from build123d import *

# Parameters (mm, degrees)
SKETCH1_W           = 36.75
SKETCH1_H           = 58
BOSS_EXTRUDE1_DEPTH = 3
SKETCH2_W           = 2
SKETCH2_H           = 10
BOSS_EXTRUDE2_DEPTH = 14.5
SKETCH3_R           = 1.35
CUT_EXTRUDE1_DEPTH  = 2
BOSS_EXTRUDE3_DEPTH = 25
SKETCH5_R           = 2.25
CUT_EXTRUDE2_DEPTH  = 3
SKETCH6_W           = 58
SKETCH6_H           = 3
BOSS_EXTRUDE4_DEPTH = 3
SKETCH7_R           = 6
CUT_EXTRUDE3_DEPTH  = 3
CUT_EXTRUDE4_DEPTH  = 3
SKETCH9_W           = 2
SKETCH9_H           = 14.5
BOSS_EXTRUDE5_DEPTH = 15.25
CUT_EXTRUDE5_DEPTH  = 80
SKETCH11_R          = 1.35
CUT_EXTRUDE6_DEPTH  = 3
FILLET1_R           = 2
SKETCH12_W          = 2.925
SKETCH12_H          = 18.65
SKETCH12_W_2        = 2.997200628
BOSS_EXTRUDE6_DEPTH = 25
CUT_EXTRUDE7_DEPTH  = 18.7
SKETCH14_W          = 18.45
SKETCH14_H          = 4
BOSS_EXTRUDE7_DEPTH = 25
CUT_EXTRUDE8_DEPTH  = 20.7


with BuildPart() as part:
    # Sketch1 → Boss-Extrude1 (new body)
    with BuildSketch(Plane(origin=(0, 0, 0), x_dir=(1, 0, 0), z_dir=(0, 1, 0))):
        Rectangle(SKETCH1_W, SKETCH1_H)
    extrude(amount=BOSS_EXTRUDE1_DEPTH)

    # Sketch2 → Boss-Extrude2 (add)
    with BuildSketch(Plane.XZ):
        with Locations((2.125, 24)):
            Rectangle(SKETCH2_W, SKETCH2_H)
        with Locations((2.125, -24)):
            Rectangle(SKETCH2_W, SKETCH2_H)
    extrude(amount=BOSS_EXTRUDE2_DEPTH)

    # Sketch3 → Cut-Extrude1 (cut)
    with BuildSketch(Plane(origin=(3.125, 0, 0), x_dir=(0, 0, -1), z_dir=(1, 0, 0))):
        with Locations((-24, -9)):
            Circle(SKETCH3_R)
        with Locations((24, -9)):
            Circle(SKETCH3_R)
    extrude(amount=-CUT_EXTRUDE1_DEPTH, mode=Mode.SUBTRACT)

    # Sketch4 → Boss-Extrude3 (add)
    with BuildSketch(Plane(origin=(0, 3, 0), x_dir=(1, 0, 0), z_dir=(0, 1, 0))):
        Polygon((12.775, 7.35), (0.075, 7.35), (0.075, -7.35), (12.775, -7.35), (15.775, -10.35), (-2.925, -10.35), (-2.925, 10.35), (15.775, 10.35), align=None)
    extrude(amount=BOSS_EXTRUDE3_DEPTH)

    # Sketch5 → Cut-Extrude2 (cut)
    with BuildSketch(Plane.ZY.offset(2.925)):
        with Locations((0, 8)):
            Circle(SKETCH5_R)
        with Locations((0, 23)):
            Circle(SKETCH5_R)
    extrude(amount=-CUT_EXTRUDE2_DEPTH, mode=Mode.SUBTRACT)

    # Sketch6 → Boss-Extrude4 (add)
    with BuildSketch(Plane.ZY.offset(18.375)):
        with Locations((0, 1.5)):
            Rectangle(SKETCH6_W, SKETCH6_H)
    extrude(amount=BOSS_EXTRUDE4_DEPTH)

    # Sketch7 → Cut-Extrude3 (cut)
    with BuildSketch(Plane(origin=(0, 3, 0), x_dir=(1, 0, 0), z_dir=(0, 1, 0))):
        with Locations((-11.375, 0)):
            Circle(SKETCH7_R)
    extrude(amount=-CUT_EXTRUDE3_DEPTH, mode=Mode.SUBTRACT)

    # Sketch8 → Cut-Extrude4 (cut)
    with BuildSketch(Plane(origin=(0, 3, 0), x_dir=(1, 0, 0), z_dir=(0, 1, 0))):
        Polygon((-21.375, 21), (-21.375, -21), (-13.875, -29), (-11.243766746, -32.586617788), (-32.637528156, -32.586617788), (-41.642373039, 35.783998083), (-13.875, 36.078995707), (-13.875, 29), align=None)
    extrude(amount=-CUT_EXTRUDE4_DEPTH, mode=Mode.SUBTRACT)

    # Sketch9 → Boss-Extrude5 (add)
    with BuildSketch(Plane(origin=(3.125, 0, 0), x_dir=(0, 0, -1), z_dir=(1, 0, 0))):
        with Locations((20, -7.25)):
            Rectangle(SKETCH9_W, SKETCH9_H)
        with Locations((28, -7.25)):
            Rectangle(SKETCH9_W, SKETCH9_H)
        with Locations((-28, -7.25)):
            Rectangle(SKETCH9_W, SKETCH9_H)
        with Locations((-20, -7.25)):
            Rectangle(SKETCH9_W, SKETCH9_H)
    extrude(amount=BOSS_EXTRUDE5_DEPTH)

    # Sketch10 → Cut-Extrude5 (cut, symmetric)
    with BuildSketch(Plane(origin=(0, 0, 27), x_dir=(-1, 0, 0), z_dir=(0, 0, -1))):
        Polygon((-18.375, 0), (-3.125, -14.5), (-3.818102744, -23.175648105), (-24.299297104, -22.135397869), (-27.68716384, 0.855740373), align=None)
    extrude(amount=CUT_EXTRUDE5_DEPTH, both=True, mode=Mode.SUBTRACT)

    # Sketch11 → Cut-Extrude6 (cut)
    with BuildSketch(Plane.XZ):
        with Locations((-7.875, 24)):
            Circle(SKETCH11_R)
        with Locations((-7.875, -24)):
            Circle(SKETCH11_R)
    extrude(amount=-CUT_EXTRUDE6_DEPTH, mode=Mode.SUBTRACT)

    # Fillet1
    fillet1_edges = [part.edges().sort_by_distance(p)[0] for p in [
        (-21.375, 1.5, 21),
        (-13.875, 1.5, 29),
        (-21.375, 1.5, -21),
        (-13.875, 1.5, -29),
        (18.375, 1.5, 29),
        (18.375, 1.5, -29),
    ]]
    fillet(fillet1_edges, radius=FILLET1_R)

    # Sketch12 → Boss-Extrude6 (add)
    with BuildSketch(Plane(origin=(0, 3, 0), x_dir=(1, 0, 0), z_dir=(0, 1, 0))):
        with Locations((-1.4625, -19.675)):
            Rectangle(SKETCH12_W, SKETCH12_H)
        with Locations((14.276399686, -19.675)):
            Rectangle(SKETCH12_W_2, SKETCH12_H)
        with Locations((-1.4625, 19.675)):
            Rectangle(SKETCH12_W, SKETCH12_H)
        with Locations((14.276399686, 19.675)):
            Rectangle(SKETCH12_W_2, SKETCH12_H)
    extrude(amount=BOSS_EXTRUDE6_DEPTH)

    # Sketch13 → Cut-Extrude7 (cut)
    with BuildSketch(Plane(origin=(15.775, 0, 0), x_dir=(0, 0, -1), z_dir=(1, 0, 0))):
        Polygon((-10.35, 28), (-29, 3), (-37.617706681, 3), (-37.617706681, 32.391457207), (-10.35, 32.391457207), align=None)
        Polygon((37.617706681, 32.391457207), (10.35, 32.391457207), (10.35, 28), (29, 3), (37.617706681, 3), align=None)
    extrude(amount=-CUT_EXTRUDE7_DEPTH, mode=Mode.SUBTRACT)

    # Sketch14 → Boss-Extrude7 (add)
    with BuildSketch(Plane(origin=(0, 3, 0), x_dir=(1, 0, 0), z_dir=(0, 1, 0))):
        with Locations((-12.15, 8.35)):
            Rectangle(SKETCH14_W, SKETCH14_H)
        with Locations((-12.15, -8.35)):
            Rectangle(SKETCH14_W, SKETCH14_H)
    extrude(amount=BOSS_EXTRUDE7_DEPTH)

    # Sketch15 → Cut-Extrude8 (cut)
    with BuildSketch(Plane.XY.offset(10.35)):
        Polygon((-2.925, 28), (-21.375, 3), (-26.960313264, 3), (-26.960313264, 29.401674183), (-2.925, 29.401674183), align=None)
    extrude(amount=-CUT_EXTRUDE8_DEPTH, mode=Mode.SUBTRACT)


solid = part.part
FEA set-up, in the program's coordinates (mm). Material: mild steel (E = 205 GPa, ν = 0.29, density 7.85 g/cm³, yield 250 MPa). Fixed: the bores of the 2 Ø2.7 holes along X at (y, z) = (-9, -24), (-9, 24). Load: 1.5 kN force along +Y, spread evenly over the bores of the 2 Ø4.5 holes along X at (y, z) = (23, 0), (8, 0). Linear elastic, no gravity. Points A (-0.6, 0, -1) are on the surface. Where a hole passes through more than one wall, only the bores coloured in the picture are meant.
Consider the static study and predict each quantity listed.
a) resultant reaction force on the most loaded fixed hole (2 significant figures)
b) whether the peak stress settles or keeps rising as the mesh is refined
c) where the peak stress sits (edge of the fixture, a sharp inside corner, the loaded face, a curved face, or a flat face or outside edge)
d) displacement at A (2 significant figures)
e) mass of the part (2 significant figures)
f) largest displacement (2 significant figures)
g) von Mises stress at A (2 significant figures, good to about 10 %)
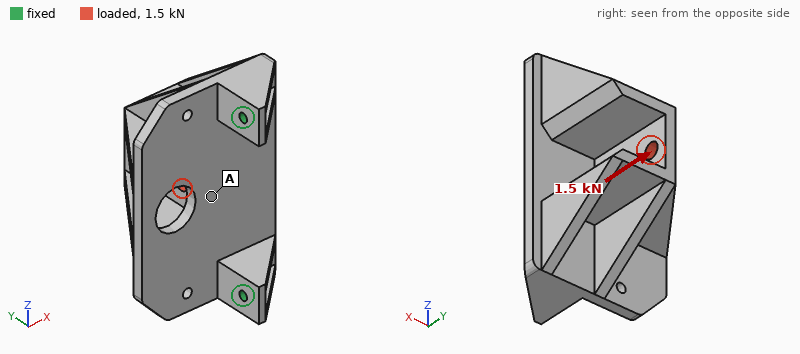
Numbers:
780 N
keeps rising
edge of the fixture
23 µm
130 g
94 µm
21 MPa
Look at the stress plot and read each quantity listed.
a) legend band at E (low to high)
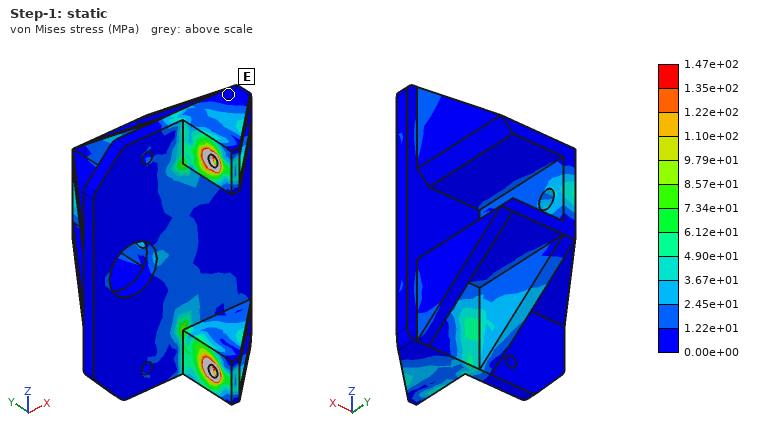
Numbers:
0.00e+00 to 1.22e+01 MPa
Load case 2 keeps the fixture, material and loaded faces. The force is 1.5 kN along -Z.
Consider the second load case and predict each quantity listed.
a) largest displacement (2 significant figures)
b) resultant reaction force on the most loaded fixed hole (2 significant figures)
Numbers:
17 µm
1000 N
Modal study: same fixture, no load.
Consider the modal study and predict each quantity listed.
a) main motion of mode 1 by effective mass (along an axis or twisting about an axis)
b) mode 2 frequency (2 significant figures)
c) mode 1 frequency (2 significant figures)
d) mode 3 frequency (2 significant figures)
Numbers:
along X
4900 Hz
1100 Hz
5000 Hz
